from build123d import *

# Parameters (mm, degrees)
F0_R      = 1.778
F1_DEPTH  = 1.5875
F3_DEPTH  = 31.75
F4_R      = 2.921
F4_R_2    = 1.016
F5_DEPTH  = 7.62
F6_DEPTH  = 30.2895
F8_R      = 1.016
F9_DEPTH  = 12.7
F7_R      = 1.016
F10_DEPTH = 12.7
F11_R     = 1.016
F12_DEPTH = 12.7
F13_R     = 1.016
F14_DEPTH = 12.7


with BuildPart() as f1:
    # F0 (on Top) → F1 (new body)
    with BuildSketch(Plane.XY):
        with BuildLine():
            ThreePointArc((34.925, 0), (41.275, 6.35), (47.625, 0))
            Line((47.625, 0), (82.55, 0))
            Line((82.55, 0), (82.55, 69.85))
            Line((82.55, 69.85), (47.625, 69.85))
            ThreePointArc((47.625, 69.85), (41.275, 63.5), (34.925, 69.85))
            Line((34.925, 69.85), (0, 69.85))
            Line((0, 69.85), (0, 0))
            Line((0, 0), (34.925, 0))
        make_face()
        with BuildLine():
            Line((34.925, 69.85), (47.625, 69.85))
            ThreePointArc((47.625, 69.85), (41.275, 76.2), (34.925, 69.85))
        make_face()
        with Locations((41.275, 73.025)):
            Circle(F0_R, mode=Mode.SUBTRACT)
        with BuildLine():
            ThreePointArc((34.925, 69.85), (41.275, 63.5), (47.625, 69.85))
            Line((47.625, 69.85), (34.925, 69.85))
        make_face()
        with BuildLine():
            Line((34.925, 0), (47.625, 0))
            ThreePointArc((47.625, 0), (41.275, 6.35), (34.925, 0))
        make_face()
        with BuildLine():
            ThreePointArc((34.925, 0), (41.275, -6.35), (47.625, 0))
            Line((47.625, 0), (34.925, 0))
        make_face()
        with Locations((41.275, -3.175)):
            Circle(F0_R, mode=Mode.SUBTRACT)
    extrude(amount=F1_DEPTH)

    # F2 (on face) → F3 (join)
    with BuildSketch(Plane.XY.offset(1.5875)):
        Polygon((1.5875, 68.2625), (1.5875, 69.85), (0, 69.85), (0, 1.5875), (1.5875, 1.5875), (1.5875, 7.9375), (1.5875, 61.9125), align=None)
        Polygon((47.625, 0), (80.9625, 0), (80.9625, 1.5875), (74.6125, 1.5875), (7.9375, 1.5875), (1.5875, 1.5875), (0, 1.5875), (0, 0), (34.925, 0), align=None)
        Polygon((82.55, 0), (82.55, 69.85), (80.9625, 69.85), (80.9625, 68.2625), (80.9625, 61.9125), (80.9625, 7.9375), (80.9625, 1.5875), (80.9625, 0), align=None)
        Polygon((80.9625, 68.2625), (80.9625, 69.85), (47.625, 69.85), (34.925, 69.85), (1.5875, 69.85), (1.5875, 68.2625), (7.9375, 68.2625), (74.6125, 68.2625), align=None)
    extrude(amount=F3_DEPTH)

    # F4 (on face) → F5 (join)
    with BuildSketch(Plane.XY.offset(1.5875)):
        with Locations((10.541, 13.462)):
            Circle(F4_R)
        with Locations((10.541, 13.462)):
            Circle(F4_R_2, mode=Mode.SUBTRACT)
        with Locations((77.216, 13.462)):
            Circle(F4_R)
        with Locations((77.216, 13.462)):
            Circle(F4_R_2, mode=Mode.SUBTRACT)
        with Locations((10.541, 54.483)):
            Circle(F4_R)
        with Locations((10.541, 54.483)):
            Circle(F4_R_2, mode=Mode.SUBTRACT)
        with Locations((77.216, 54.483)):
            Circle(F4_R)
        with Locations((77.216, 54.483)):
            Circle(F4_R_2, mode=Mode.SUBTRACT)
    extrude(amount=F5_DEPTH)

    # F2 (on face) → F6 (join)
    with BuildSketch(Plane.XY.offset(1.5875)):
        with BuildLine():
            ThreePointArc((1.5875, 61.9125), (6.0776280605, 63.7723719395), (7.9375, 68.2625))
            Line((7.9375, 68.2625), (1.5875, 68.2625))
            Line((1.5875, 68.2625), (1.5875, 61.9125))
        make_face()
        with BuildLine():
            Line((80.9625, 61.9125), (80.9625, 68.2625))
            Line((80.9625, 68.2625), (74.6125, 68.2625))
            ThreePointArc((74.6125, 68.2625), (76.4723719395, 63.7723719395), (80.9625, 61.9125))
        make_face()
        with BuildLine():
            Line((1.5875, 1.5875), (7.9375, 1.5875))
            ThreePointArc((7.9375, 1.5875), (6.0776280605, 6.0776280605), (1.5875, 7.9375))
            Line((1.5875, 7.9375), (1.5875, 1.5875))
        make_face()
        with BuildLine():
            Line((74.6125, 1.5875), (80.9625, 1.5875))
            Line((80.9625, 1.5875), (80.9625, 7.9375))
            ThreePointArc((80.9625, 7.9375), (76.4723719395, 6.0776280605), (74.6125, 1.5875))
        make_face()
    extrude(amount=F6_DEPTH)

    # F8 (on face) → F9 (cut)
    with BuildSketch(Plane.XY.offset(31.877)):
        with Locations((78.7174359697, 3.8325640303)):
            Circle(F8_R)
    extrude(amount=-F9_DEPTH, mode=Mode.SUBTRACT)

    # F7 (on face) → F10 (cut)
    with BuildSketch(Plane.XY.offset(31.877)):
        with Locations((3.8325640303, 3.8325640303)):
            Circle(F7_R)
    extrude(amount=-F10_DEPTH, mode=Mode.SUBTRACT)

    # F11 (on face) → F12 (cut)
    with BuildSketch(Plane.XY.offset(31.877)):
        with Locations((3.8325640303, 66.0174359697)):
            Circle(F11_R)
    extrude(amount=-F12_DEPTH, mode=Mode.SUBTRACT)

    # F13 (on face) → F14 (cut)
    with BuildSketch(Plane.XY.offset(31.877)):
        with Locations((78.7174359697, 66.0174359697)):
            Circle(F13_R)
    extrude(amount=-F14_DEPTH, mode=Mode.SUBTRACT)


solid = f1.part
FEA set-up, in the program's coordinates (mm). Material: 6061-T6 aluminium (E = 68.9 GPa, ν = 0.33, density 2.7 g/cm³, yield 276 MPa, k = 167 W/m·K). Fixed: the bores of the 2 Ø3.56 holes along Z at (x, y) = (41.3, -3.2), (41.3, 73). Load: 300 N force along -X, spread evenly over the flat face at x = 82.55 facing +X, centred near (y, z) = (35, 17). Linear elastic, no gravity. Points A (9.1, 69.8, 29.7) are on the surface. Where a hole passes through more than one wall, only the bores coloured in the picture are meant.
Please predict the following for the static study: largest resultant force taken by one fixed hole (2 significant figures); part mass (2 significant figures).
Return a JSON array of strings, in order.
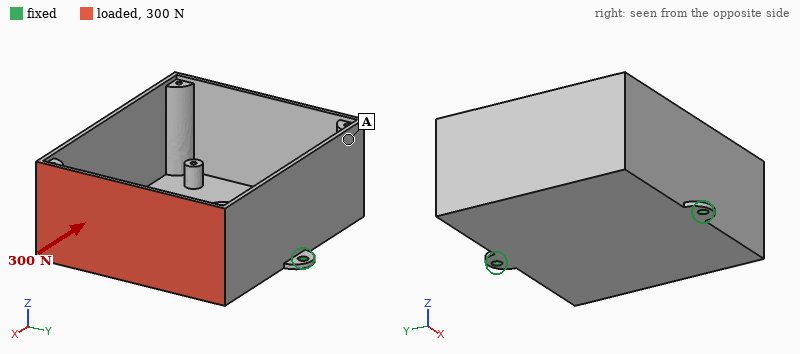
["150 N", "78 g"]
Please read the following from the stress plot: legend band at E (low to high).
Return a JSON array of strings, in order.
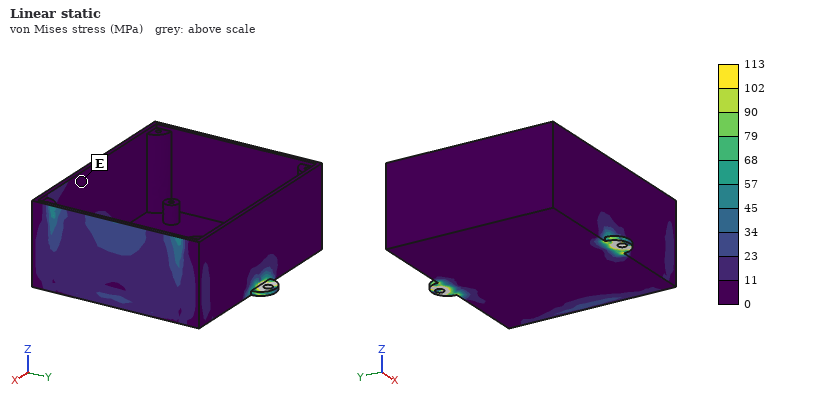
["0 to 11 MPa"]
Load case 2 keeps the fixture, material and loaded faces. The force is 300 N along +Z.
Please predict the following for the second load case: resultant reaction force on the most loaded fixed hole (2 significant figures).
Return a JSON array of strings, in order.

["150 N"]
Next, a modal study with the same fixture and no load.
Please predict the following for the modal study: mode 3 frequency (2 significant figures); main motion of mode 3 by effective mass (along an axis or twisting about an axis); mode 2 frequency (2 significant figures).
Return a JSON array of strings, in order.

["1900 Hz", "along Z", "720 Hz"]
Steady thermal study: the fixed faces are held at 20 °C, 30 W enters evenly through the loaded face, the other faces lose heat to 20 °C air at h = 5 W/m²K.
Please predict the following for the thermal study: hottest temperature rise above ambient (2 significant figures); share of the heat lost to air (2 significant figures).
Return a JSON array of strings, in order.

["67 K", "16 %"]
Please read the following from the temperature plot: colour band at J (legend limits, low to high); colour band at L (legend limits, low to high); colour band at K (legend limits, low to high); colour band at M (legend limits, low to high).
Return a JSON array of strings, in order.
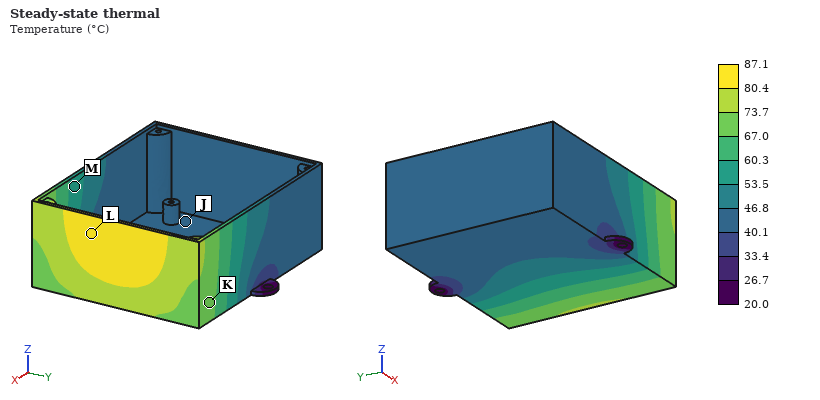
["40.1 to 46.8 °C", "80.4 to 87.1 °C", "67.0 to 73.7 °C", "53.5 to 60.3 °C"]
